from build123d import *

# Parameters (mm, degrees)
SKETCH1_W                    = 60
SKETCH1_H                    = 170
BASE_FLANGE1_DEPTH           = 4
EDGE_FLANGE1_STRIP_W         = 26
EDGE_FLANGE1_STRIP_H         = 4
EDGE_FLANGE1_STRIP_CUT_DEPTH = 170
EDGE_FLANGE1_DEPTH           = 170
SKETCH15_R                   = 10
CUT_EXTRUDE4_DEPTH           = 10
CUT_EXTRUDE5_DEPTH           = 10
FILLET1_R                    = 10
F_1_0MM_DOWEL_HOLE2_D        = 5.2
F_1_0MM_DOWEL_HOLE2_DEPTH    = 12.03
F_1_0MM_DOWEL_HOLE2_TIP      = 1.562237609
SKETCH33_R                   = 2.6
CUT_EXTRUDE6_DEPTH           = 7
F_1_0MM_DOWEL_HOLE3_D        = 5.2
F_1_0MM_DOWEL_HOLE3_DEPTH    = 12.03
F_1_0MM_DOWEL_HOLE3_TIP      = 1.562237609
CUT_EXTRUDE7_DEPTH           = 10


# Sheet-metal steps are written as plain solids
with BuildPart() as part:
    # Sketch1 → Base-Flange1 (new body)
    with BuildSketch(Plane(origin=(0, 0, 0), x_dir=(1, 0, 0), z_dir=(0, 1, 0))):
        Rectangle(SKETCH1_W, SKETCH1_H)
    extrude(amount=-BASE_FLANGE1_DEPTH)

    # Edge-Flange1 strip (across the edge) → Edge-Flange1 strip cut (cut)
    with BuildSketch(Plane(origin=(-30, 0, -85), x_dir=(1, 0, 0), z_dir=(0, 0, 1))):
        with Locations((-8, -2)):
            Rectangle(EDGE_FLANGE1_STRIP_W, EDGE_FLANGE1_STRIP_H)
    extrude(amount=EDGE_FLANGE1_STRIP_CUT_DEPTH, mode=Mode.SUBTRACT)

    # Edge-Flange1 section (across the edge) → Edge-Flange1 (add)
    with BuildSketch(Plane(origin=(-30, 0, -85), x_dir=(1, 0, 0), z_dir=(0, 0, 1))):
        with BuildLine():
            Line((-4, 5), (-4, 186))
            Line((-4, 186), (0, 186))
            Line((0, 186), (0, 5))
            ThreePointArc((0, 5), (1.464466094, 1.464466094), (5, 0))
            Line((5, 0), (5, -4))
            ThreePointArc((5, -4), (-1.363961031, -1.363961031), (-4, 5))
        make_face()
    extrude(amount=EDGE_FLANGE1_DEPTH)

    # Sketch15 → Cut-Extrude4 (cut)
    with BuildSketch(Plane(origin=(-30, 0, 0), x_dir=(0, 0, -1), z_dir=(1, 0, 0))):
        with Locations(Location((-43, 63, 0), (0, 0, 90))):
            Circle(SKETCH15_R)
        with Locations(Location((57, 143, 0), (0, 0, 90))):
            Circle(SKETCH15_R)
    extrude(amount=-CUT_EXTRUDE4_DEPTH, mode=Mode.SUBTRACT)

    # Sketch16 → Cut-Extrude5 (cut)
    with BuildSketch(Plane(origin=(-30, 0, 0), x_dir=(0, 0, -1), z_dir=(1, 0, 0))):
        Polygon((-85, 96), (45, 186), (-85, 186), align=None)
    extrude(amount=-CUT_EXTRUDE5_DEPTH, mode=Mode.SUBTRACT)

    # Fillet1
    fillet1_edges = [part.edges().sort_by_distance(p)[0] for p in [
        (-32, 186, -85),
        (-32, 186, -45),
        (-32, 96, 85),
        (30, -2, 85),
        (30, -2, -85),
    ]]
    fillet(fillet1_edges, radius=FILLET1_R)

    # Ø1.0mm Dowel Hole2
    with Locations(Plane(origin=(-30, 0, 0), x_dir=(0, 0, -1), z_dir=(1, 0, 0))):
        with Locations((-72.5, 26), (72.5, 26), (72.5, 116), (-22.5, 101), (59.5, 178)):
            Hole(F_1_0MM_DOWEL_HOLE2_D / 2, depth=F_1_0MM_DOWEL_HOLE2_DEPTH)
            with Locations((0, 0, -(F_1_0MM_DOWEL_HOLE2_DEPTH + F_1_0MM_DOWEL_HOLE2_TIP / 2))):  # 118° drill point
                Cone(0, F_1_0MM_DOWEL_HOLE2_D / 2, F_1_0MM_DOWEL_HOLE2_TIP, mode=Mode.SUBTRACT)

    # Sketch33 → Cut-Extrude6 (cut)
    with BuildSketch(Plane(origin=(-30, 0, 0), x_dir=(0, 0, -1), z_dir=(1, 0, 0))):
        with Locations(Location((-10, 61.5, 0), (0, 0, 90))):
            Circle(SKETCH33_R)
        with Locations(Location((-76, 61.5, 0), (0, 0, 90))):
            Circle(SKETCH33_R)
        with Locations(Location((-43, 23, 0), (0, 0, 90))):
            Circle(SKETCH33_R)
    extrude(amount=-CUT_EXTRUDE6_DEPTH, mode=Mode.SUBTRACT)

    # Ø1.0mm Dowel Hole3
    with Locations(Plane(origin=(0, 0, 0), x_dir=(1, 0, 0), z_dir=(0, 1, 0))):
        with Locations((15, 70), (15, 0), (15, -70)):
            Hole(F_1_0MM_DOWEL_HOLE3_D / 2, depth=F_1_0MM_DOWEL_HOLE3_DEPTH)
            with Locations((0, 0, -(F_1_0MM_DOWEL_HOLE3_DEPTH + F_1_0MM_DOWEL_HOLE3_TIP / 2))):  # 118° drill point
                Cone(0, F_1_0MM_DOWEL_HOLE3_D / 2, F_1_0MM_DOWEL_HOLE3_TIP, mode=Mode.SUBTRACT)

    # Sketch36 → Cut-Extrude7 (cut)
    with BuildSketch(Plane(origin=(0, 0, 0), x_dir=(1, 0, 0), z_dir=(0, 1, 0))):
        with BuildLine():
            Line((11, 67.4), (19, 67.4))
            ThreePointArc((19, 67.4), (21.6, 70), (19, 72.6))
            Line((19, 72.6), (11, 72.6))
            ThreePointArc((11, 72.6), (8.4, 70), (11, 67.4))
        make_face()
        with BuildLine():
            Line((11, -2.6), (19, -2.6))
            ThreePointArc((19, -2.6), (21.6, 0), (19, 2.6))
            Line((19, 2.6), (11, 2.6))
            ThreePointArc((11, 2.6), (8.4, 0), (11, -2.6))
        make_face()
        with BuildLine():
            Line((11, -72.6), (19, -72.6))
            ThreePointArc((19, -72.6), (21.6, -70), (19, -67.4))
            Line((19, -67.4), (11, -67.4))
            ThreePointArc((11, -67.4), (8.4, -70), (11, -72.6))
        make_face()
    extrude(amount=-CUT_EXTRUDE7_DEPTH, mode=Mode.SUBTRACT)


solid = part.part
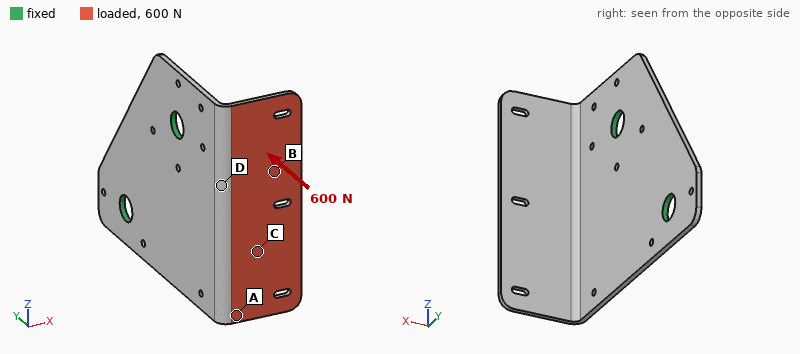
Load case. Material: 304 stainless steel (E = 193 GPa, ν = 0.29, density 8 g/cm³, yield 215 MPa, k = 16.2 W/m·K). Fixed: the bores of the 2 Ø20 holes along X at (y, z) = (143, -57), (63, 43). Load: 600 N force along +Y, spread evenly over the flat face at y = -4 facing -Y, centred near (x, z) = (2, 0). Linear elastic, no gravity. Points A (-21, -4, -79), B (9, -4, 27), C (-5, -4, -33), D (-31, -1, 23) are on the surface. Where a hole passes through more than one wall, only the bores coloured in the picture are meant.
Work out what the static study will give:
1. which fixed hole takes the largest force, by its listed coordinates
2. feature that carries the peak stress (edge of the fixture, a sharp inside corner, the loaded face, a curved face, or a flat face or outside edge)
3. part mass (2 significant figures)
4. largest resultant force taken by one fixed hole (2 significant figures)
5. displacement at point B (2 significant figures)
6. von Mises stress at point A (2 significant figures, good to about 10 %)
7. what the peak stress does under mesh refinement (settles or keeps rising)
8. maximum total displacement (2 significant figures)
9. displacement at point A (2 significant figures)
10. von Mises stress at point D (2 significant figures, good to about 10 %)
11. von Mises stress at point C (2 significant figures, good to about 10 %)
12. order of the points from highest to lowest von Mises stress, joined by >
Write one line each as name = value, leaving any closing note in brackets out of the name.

which fixed hole takes the largest force, by its listed coordinates = (63, 43)
feature that carries the peak stress = edge of the fixture
part mass = 1.1 kg
largest resultant force taken by one fixed hole = 360 N
displacement at point B = 0.48 mm
von Mises stress at point A = 24 MPa
what the peak stress does under mesh refinement = keeps rising
maximum total displacement = 0.74 mm
displacement at point A = 0.45 mm
von Mises stress at point D = 30 MPa
von Mises stress at point C = 12 MPa
order of the points from highest to lowest von Mises stress, joined by > = D > A > C > B
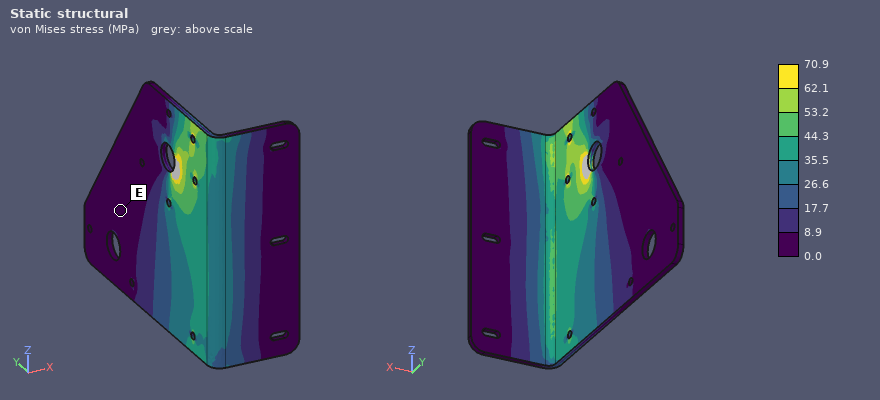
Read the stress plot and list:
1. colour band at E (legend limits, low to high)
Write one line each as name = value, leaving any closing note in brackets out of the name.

colour band at E = 0.0 to 8.9 MPa
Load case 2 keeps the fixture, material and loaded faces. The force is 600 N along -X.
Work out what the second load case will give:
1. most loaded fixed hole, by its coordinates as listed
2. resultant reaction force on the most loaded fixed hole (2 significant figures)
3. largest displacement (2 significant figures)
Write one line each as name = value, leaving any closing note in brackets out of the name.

most loaded fixed hole, by its coordinates as listed = (63, 43)
resultant reaction force on the most loaded fixed hole = 590 N
largest displacement = 1.2 mm
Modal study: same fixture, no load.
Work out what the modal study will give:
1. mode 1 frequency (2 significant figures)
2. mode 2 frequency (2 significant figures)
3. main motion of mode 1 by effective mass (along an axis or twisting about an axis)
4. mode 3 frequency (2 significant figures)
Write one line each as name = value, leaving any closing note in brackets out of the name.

mode 1 frequency = 200 Hz
mode 2 frequency = 350 Hz
main motion of mode 1 by effective mass = along X
mode 3 frequency = 630 Hz
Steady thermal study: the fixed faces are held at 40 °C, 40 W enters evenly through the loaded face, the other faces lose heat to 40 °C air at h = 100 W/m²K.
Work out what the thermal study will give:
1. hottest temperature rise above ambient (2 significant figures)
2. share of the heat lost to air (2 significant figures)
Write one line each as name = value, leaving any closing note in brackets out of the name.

hottest temperature rise above ambient = 34 K
share of the heat lost to air = 100 %
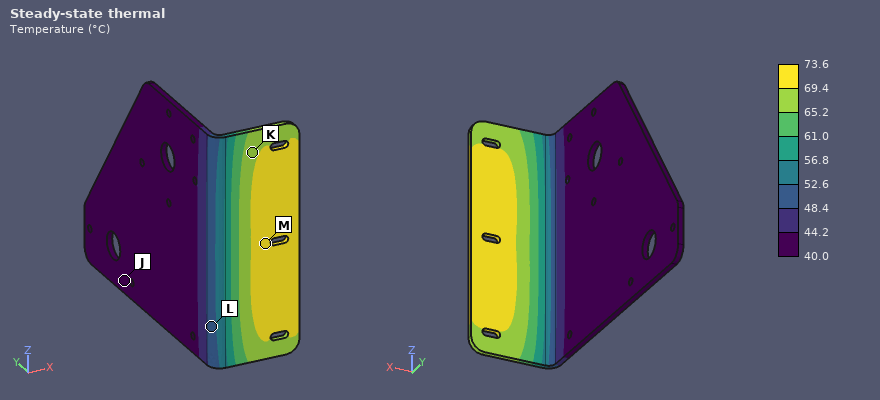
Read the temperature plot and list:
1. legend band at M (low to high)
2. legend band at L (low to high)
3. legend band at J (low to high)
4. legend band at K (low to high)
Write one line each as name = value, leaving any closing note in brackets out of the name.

legend band at M = 69.4 to 73.6 °C
legend band at L = 48.4 to 52.6 °C
legend band at J = 40.0 to 44.2 °C
legend band at K = 65.2 to 69.4 °C
